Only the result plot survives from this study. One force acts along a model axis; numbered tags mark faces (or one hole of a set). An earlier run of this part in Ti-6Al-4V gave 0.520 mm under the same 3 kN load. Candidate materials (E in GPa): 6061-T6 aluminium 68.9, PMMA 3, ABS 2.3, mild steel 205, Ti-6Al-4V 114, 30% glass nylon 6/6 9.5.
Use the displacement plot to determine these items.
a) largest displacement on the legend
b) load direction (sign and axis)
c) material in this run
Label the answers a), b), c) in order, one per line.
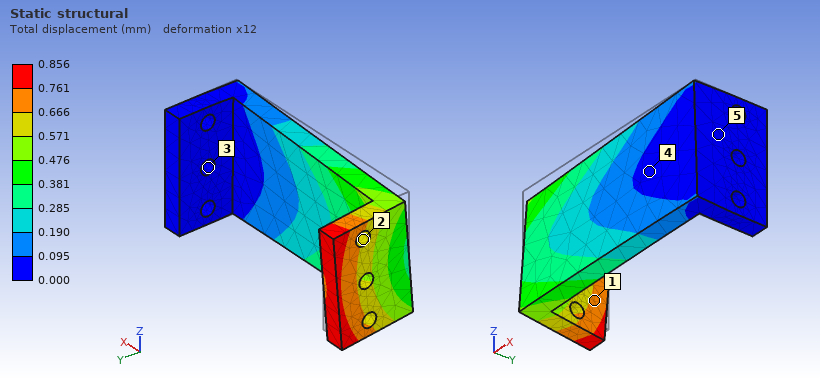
a) 0.856 mm
b) -Z
c) 6061-T6 aluminium
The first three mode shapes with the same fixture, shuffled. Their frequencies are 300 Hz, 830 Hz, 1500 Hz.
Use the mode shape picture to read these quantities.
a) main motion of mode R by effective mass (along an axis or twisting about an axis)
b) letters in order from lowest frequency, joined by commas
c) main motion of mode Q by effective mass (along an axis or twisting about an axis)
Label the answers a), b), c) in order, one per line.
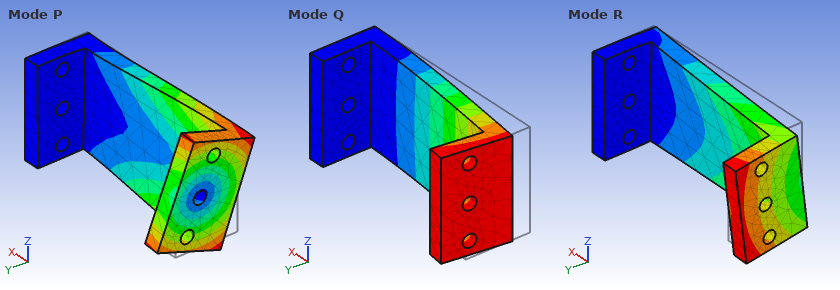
a) along Z
b) Q, R, P
c) along Y
